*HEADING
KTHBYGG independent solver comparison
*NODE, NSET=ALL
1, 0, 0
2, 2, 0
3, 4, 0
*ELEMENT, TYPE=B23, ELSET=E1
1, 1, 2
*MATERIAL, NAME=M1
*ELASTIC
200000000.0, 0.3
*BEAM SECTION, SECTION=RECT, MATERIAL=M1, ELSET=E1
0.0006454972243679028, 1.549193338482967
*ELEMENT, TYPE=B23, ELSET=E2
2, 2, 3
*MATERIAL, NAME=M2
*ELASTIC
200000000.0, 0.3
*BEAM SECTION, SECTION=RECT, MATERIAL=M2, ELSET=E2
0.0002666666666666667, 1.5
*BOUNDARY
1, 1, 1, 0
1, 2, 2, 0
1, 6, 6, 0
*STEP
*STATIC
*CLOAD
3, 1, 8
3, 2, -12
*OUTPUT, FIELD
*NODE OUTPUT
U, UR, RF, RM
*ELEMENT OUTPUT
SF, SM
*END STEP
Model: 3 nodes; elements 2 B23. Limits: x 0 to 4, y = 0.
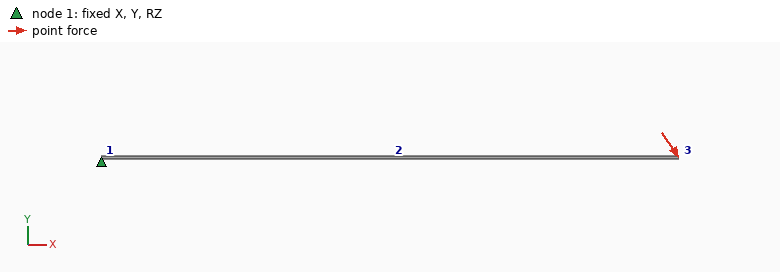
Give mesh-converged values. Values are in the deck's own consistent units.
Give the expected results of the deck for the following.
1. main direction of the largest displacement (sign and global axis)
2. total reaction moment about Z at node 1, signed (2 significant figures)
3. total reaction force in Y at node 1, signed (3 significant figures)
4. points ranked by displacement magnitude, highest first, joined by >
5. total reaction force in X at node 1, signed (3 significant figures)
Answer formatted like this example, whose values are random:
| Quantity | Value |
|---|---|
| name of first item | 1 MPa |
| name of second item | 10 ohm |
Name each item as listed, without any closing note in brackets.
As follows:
| Quantity | Value |
|---|---|
| main direction of the largest displacement | -Y |
| total reaction moment about Z at node 1, signed | 48 |
| total reaction force in Y at node 1, signed | 12.0 |
| points ranked by displacement magnitude, highest first, joined by > | node 3 > node 2 > node 1 |
| total reaction force in X at node 1, signed | -8.00 |
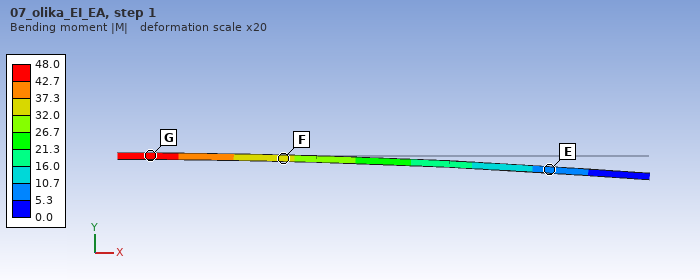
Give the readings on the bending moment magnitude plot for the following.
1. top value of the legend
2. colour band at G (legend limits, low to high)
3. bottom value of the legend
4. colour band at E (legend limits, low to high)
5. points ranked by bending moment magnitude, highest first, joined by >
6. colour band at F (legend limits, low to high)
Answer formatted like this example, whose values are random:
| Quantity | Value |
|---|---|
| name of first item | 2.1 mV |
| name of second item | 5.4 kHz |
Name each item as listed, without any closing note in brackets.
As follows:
| Quantity | Value |
|---|---|
| top value of the legend | 48.0 |
| colour band at G | 42.7 to 48.0 |
| bottom value of the legend | 0.0 |
| colour band at E | 5.3 to 10.7 |
| points ranked by bending moment magnitude, highest first, joined by > | G > F > E |
| colour band at F | 32.0 to 37.3 |
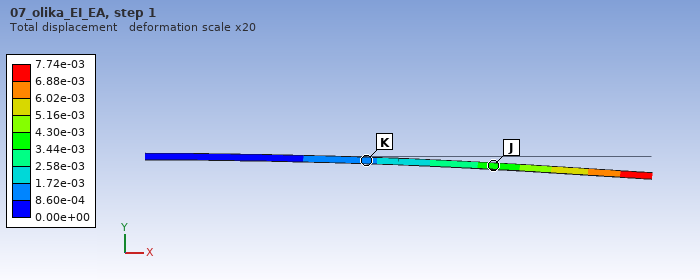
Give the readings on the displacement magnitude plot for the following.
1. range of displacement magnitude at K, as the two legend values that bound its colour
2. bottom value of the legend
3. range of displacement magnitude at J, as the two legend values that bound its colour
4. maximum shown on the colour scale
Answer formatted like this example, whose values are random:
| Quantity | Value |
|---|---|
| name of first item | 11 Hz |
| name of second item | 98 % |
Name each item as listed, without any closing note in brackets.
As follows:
| Quantity | Value |
|---|---|
| range of displacement magnitude at K, as the two legend values that bound its colour | 8.60e-04 to 1.72e-03 |
| bottom value of the legend | 0.00e+00 |
| range of displacement magnitude at J, as the two legend values that bound its colour | 3.44e-03 to 4.30e-03 |
| maximum shown on the colour scale | 7.74e-03 |
